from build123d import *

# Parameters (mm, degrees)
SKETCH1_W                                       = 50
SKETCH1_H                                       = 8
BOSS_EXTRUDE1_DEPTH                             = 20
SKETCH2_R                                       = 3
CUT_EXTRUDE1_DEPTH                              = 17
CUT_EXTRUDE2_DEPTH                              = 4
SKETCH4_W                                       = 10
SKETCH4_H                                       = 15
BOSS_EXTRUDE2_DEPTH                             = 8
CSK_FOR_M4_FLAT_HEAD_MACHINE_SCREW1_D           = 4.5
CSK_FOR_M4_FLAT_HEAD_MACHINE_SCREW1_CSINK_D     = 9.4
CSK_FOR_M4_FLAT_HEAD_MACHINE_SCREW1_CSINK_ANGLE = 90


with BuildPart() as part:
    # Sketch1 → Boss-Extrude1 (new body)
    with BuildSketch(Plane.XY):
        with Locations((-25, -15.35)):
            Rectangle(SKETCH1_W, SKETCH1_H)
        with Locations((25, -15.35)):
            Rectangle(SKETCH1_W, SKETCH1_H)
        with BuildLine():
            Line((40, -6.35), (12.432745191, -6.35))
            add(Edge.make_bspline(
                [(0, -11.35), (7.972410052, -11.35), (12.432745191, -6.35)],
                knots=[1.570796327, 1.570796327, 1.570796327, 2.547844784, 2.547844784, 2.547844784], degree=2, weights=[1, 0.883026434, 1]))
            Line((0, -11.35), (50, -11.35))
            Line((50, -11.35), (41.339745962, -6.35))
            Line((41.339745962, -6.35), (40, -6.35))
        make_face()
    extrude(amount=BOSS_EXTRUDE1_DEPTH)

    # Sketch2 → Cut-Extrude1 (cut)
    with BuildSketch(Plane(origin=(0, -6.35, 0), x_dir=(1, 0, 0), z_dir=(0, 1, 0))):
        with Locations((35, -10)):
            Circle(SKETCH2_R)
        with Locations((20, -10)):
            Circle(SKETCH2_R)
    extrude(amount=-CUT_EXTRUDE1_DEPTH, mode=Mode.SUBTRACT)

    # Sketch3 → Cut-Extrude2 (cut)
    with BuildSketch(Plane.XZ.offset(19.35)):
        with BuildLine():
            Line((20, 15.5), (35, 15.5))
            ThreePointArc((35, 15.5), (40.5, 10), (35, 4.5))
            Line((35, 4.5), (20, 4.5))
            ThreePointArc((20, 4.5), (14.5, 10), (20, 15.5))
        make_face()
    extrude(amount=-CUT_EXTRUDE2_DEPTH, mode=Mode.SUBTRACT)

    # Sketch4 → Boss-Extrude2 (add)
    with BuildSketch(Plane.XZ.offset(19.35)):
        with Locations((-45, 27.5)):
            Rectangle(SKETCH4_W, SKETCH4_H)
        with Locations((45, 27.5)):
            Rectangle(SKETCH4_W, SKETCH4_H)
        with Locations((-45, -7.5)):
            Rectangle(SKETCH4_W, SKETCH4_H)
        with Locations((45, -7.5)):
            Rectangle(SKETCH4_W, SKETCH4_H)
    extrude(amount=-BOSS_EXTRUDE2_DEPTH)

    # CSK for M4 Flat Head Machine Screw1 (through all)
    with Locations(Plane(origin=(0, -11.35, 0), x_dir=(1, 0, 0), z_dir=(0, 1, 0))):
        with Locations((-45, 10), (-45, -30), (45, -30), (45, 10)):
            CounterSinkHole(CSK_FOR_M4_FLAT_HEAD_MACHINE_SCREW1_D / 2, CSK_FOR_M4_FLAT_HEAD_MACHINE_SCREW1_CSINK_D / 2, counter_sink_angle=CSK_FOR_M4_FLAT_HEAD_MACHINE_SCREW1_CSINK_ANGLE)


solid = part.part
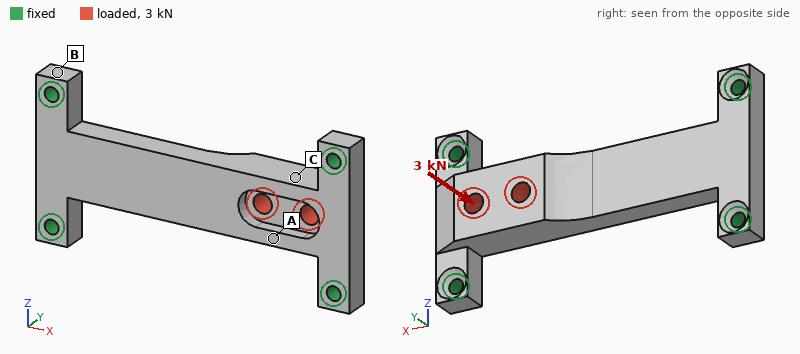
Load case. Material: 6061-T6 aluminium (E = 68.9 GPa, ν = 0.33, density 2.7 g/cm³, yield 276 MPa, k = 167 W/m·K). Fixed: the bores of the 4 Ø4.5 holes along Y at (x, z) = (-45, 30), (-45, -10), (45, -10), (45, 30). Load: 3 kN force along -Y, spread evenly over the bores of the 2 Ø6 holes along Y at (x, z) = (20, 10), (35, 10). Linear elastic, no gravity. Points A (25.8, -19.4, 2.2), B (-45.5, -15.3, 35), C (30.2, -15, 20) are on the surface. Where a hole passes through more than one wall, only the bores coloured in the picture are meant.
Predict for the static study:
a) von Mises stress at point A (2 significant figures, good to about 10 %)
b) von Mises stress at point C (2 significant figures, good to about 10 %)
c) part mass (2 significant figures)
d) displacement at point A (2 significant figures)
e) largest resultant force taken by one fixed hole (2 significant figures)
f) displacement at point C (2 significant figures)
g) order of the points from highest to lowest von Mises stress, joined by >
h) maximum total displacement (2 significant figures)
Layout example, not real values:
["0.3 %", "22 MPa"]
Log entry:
["52 MPa", "28 MPa", "60 g", "0.10 mm", "1.5 kN", "0.083 mm", "A > C > B", "0.15 mm"]
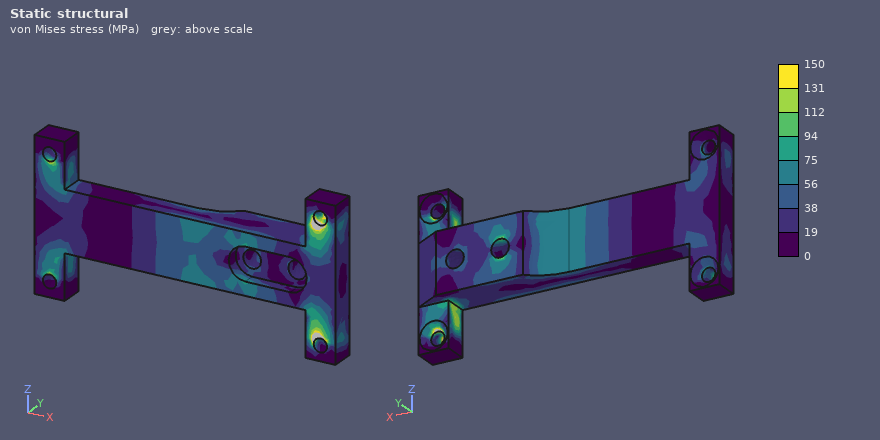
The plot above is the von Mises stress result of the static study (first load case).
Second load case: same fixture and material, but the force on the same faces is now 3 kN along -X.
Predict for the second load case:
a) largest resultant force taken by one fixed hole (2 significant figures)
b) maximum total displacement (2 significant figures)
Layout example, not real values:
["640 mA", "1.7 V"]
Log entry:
["920 N", "36 µm"]
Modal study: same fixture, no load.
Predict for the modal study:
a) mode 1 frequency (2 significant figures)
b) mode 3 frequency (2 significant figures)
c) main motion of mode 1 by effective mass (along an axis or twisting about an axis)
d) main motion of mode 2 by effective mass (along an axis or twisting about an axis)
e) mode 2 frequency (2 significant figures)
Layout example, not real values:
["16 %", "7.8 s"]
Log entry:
["3400 Hz", "10 kHz", "along Y", "along Z", "8100 Hz"]
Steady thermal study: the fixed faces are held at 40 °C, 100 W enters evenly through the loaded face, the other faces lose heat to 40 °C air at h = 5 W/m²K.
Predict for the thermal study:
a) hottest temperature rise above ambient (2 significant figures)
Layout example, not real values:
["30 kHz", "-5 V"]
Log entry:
["66 K"]
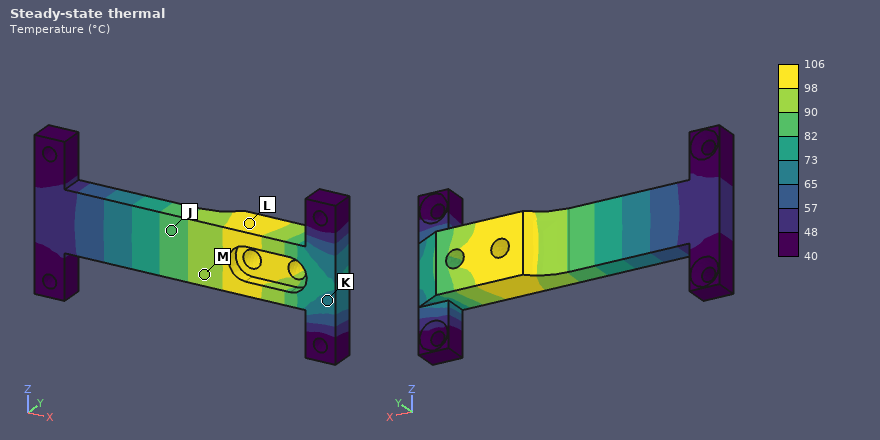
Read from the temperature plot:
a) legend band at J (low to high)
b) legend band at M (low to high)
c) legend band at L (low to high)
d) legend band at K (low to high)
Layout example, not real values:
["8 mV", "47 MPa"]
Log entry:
["82 to 90 °C", "90 to 98 °C", "98 to 106 °C", "65 to 73 °C"]
